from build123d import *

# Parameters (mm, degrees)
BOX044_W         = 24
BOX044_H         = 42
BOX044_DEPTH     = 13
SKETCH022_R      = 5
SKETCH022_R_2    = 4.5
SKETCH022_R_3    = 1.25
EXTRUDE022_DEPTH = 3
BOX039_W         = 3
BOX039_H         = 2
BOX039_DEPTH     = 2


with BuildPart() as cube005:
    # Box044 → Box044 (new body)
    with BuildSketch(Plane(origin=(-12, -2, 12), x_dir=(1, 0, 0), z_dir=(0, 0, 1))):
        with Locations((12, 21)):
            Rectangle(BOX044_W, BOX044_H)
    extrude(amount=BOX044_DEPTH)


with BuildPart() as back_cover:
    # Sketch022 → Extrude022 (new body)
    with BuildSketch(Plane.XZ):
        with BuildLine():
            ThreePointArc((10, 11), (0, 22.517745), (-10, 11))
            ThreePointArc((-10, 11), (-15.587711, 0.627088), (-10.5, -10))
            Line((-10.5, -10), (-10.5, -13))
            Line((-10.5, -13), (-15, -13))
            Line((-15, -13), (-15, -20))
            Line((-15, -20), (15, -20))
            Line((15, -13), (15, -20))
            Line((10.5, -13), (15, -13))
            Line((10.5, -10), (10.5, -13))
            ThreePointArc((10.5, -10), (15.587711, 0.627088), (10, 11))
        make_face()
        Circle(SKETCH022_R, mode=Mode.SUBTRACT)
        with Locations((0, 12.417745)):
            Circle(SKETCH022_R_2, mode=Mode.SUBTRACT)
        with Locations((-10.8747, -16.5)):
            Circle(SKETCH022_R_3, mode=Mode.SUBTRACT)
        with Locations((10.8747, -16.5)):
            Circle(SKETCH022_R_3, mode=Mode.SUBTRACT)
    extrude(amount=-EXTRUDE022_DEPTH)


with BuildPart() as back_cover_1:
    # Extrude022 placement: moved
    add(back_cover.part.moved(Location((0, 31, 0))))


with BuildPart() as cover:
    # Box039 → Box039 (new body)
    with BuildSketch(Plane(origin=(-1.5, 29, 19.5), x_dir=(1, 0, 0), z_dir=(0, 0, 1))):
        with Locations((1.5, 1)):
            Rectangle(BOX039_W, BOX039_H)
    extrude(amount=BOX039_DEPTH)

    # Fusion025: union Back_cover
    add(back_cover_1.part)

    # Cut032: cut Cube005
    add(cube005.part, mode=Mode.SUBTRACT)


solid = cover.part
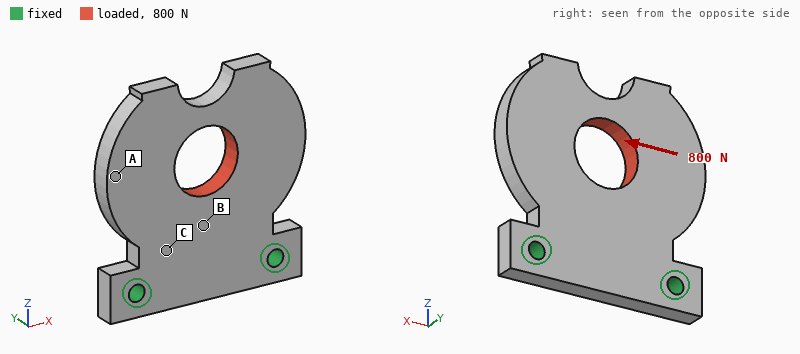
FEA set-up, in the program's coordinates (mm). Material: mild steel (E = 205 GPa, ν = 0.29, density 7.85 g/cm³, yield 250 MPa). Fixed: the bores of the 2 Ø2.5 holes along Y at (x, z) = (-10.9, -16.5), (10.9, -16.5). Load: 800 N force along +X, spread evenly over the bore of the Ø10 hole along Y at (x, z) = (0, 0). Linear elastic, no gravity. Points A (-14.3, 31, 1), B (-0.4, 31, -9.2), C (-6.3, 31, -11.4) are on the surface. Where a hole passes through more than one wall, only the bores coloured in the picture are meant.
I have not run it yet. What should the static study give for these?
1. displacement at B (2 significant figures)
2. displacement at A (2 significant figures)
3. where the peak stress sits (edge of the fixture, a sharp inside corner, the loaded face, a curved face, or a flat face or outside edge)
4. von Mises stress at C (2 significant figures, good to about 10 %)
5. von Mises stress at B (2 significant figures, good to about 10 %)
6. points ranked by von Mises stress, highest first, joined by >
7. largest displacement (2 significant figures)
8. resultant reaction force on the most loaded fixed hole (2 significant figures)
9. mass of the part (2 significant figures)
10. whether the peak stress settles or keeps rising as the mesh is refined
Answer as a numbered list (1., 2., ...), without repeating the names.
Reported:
1. 1.9 µm
2. 8.3 µm
3. a sharp inside corner
4. 27 MPa
5. 40 MPa
6. B > C > A
7. 12 µm
8. 740 N
9. 18 g
10. keeps rising
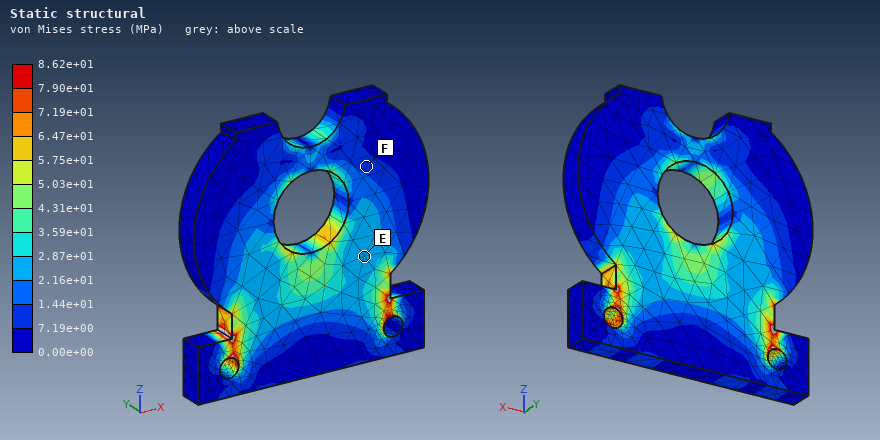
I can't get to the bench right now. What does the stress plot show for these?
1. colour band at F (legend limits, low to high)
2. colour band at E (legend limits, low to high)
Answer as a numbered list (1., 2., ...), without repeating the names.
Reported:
1. 7.19e+00 to 1.44e+01 MPa
2. 2.16e+01 to 2.87e+01 MPa
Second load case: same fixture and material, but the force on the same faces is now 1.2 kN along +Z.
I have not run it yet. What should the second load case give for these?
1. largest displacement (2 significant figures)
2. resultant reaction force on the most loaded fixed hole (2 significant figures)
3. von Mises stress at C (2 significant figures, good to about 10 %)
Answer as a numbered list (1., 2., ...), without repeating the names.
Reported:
1. 4.6 µm
2. 630 N
3. 22 MPa
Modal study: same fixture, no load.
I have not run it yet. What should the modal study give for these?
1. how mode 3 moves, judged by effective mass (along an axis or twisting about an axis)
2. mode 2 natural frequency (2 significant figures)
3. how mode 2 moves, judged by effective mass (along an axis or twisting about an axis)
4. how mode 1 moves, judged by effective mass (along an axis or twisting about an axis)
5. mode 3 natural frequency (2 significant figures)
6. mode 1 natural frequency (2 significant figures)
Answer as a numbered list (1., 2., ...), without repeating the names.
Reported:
1. along X
2. 6100 Hz
3. twisting about Z
4. along Y
5. 14 kHz
6. 2700 Hz
